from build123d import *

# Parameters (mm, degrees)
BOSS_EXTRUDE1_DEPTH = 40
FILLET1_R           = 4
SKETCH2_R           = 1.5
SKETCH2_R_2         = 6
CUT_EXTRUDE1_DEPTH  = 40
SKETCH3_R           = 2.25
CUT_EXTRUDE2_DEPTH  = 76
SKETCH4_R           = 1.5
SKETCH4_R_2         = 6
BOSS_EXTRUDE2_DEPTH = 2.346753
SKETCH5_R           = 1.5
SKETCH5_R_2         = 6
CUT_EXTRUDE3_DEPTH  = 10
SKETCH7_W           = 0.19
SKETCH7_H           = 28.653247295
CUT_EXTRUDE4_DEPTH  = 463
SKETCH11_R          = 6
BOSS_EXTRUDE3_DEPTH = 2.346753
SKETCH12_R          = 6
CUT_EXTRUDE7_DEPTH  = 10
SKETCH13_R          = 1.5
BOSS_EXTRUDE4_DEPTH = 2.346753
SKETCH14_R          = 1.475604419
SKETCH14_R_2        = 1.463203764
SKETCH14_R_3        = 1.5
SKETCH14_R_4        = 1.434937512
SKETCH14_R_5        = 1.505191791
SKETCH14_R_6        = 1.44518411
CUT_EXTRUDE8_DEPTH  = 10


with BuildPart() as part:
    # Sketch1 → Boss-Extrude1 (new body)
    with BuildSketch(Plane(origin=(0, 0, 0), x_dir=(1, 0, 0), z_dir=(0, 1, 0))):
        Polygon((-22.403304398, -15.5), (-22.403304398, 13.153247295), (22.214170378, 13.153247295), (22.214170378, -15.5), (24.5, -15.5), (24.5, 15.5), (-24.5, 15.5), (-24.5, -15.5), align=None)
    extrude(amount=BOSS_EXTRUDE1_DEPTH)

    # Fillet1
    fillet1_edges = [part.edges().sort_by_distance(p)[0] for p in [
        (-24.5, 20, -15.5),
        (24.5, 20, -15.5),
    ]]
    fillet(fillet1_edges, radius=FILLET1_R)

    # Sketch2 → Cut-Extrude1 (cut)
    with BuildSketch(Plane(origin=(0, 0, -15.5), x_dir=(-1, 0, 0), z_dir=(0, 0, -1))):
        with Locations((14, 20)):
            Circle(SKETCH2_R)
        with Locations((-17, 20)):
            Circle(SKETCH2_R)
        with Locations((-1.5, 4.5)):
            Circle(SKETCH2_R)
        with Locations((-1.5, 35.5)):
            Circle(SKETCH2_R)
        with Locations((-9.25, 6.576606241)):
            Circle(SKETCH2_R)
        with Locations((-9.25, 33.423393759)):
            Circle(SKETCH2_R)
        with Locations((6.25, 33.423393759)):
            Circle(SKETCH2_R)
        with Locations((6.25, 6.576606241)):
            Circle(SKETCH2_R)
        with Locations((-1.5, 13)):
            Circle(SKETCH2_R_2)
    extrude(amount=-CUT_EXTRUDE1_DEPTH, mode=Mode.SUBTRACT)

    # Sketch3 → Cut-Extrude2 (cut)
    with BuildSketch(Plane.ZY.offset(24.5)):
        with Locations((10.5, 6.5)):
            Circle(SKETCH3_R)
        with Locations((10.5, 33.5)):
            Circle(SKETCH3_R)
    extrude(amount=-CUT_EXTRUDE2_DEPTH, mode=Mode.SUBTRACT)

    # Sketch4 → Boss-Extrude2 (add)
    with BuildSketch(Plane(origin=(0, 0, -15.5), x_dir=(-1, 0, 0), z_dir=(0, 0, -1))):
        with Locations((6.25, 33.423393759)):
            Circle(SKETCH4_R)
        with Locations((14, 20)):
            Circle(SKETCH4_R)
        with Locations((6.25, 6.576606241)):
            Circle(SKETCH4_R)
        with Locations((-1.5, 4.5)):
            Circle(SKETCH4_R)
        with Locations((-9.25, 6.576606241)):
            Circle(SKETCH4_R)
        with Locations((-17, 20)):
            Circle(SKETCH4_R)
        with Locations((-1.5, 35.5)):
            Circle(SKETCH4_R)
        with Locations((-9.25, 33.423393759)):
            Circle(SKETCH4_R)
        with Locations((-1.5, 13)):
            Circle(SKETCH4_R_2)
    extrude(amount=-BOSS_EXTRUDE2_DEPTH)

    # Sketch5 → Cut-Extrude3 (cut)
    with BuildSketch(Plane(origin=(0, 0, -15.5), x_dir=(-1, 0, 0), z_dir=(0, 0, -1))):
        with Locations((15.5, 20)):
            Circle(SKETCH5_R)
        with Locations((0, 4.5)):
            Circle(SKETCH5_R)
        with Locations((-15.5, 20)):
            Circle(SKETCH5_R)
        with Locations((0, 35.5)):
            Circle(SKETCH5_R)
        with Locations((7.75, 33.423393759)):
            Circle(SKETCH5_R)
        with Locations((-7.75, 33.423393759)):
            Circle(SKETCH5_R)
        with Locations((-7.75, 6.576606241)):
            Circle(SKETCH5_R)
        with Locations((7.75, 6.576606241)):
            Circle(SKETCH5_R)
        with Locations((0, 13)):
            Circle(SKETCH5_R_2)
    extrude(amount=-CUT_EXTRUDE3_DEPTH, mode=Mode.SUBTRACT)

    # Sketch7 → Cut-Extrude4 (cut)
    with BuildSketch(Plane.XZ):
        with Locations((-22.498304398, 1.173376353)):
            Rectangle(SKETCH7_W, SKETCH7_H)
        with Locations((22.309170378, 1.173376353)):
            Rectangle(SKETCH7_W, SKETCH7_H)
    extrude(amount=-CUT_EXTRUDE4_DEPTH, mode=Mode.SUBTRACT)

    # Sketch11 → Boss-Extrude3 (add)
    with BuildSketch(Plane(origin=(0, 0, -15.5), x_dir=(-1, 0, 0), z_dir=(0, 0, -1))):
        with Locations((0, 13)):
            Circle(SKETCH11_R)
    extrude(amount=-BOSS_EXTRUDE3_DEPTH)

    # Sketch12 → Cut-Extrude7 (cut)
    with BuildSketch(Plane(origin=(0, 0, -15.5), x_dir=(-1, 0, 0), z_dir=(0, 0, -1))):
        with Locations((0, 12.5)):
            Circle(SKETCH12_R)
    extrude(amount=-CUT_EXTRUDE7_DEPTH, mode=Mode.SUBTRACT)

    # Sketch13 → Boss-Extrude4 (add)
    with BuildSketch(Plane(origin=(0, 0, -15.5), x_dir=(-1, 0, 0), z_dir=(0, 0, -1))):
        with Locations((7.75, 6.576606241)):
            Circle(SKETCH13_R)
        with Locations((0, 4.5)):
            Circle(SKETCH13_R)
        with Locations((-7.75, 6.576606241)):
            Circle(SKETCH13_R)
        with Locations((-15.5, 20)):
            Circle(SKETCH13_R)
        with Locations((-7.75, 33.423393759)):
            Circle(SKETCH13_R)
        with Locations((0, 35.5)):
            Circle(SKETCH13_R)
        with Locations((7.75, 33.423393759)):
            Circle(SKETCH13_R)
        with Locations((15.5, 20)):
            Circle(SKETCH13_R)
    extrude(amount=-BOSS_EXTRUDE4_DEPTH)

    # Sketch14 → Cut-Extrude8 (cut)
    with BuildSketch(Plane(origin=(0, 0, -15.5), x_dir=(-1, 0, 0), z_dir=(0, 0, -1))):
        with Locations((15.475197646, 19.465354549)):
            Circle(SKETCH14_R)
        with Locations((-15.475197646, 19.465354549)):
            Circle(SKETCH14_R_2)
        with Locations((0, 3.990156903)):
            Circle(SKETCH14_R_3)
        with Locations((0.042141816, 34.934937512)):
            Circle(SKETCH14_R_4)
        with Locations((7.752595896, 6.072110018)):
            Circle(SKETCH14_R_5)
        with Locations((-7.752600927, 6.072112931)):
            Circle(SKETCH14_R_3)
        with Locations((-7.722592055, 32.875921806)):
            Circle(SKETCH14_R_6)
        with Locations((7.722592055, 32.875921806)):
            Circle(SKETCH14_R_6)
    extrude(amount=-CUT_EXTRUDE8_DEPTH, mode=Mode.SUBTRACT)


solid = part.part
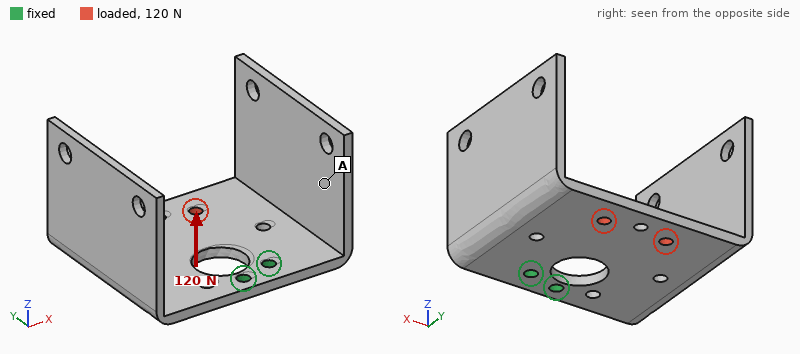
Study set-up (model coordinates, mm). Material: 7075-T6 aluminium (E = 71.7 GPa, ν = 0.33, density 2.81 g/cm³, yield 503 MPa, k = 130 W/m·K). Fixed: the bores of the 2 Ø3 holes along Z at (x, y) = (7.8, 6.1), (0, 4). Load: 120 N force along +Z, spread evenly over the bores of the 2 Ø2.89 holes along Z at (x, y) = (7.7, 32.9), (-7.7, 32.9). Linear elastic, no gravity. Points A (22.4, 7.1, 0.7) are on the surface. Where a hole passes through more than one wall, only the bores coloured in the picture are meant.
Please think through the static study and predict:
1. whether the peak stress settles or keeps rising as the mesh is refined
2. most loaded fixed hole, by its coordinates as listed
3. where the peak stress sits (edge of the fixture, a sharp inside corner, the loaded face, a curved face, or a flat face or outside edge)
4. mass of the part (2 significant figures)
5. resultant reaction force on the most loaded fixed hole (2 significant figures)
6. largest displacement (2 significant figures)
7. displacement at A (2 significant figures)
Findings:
keeps rising
(7.8, 6.1)
edge of the fixture
24 g
98 N
0.81 mm
0.17 mm
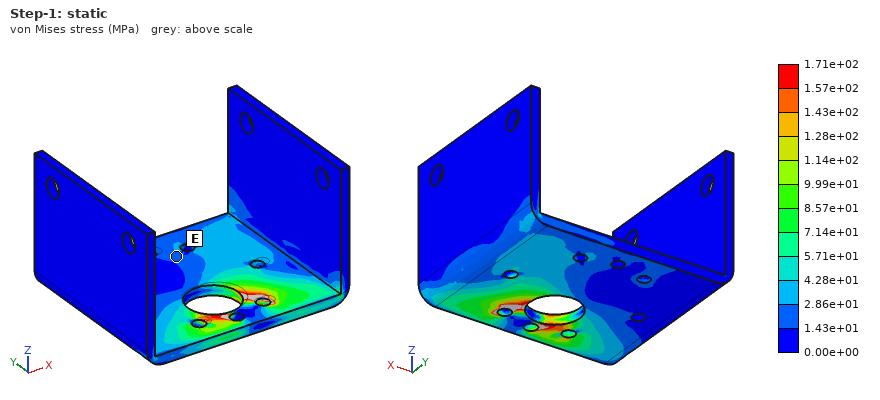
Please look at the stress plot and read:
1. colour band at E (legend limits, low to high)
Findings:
1.43e+01 to 2.86e+01 MPa
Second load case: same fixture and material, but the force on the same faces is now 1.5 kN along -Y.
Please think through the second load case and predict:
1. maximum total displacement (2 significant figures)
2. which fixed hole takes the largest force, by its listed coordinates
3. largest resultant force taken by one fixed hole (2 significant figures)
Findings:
94 µm
(0, 4)
1.0 kN
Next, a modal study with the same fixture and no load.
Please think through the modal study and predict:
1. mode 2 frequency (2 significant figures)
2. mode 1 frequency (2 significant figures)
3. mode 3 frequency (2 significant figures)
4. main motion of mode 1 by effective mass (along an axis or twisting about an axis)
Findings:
790 Hz
580 Hz
1000 Hz
along Z
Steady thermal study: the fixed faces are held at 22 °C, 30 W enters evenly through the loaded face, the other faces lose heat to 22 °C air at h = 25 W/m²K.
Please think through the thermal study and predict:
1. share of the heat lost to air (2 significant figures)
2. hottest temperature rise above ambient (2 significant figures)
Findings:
31 %
83 K
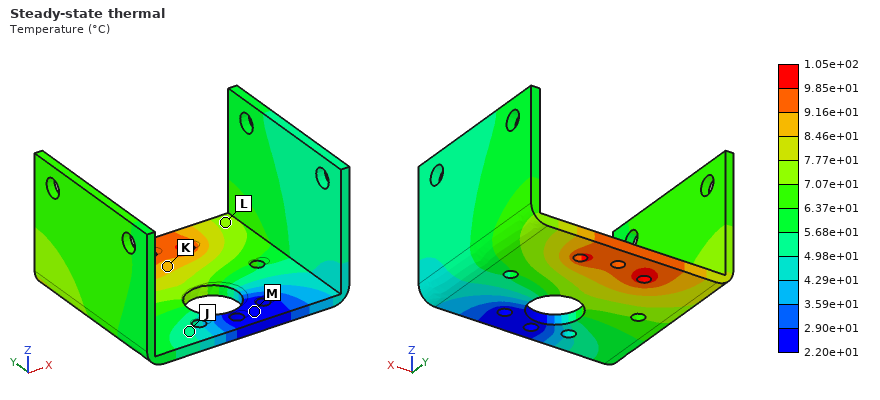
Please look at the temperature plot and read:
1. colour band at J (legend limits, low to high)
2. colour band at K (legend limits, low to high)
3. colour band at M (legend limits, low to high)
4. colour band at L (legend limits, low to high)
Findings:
4.98e+01 to 5.68e+01 °C
8.46e+01 to 9.16e+01 °C
2.20e+01 to 2.90e+01 °C
7.07e+01 to 7.77e+01 °C
